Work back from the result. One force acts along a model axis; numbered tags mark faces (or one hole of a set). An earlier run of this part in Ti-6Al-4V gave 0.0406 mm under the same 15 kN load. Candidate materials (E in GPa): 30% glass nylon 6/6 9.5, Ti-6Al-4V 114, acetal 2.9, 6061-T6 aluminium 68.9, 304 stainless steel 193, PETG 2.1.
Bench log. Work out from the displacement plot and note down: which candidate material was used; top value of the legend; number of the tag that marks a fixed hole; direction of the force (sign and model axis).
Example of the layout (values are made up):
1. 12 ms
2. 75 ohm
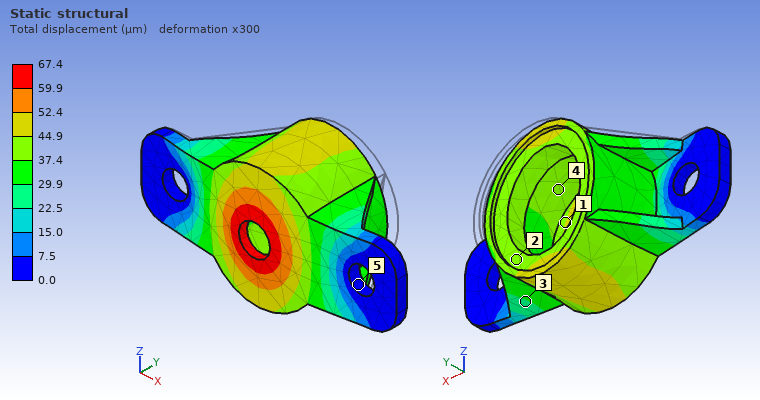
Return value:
1. 6061-T6 aluminium
2. 67.4 µm
3. 5
4. -Y
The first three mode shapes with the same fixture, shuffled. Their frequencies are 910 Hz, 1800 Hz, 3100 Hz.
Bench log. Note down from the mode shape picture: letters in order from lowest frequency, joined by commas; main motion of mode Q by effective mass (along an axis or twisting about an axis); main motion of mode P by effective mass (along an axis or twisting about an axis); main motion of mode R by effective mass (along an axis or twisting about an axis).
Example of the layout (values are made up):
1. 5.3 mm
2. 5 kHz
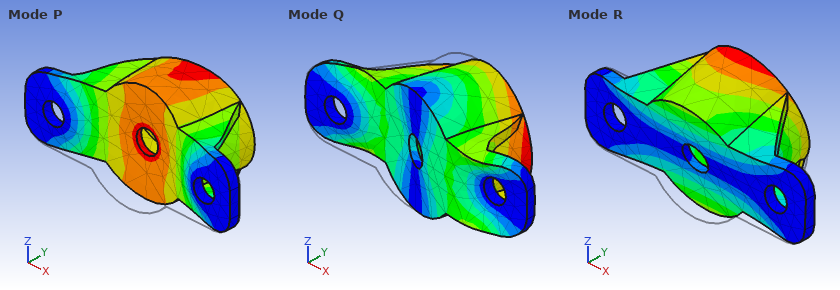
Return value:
1. R, P, Q
2. along X
3. along Y
4. along Z
